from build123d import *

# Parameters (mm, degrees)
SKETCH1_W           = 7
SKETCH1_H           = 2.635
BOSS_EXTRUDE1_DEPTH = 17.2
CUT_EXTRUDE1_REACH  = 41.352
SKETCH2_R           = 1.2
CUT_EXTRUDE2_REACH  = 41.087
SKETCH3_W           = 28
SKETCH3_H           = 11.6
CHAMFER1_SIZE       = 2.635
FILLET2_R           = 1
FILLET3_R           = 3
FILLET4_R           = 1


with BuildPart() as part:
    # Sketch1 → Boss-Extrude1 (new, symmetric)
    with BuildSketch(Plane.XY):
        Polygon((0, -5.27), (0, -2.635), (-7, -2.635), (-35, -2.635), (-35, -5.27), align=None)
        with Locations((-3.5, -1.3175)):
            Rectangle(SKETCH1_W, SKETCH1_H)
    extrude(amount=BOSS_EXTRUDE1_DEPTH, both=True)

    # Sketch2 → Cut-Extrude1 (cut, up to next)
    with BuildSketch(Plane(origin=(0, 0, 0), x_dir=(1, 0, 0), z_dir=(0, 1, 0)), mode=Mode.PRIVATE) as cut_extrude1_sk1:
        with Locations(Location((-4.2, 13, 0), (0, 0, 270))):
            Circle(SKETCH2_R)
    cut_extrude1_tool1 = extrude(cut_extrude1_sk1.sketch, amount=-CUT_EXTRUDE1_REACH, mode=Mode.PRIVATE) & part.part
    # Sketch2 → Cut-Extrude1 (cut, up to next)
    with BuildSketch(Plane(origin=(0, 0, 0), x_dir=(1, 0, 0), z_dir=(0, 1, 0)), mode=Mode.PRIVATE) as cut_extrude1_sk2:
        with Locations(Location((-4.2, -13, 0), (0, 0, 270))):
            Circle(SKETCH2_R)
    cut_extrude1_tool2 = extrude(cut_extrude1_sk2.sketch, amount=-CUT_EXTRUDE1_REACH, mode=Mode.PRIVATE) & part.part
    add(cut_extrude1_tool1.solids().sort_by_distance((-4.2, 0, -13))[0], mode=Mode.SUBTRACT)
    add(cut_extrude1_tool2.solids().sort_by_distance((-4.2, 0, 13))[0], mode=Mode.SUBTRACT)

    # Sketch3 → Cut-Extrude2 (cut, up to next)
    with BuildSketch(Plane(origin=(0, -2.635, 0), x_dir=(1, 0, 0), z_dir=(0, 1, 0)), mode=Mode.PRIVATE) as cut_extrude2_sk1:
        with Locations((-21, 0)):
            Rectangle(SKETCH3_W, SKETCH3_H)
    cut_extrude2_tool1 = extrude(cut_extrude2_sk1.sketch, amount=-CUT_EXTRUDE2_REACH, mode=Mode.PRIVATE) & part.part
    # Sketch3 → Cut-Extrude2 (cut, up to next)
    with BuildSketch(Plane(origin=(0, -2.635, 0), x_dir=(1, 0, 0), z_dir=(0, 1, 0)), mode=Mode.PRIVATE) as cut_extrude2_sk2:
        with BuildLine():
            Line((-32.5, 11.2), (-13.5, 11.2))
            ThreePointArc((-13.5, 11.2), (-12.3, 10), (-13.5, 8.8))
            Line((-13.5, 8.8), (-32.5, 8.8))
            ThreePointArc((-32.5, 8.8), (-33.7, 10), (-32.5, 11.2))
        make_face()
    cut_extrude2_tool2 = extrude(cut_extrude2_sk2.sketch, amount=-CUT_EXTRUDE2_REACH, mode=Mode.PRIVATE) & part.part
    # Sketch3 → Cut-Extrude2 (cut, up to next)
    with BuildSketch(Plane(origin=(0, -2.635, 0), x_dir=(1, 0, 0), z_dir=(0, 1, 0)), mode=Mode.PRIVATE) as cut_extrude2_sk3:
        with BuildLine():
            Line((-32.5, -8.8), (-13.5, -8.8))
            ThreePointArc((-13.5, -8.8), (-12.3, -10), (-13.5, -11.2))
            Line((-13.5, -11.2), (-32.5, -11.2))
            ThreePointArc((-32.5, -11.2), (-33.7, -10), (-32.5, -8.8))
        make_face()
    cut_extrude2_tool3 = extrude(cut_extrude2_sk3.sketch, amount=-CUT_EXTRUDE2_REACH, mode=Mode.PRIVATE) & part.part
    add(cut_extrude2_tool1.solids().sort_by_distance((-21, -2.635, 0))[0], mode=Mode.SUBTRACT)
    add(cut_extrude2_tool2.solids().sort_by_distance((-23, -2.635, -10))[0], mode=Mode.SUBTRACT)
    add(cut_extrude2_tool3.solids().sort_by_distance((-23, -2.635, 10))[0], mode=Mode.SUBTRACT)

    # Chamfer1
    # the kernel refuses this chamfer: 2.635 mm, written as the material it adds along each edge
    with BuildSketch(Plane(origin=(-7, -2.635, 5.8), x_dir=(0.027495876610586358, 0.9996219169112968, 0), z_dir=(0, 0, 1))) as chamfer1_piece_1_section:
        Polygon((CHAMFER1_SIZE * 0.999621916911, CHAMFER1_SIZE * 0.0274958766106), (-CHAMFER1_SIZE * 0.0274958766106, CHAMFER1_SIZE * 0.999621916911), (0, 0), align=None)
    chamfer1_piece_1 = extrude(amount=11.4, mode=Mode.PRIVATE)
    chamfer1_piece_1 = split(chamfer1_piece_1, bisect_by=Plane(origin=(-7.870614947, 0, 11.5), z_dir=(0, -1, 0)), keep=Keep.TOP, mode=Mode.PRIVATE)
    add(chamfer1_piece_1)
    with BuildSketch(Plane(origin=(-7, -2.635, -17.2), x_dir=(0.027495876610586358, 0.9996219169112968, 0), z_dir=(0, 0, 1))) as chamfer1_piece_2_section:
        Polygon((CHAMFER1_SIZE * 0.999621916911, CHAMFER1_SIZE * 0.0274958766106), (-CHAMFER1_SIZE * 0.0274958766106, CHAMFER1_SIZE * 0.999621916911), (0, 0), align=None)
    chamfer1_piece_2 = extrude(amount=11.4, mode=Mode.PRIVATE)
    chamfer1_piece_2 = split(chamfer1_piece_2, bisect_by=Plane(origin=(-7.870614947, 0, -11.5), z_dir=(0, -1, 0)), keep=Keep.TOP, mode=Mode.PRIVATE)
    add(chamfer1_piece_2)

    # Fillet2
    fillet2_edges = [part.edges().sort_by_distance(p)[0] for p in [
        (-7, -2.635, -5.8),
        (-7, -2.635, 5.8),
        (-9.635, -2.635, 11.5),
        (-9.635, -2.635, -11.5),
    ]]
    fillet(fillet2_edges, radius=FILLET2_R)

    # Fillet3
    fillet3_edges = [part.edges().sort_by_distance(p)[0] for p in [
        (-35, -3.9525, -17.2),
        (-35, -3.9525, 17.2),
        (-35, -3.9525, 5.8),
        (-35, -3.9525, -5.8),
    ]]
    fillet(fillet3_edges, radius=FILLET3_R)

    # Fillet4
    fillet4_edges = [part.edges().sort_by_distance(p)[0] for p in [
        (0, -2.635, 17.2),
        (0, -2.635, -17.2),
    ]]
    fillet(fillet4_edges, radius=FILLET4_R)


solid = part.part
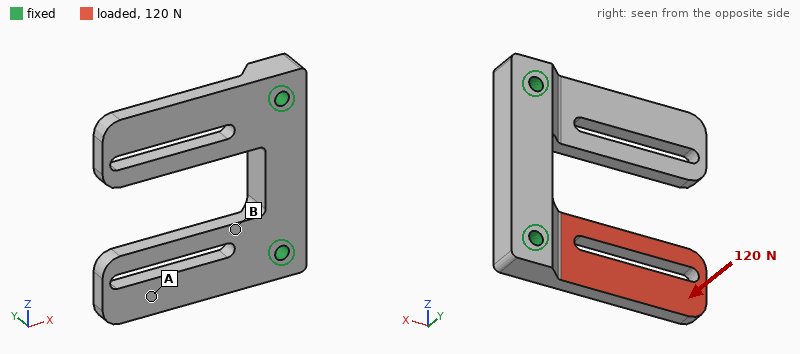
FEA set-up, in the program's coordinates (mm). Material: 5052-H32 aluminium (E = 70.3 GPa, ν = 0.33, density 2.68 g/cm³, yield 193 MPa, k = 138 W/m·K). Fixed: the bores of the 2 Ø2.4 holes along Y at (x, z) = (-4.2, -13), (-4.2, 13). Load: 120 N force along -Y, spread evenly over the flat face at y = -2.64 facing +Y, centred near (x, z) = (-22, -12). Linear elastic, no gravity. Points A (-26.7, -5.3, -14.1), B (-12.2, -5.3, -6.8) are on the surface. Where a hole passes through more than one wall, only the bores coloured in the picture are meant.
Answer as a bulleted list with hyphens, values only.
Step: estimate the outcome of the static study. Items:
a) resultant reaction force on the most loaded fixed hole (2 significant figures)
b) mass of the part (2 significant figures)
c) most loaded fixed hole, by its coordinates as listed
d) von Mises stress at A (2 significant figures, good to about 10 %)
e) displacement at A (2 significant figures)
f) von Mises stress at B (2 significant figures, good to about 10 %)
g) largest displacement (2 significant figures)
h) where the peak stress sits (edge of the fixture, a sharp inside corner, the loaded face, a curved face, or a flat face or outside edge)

- 130 N
- 7.2 g
- (-4.2, -13)
- 15 MPa
- 0.18 mm
- 100 MPa
- 0.31 mm
- the loaded face
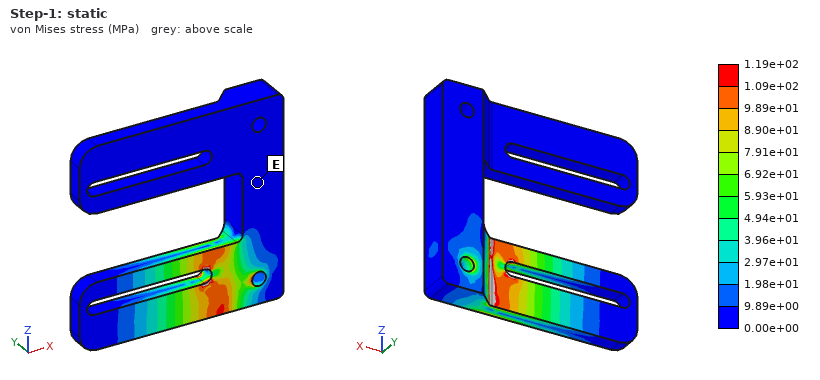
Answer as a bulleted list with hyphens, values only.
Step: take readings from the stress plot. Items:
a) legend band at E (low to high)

- 0.00e+00 to 9.89e+00 MPa
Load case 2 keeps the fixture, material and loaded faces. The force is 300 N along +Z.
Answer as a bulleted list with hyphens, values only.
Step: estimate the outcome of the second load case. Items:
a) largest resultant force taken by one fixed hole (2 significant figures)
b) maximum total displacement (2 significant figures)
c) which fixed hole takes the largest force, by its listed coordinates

- 330 N
- 0.15 mm
- (-4.2, -13)
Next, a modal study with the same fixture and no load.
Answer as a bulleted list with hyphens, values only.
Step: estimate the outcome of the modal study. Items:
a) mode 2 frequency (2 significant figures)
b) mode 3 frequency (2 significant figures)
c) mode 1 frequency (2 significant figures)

- 3100 Hz
- 6600 Hz
- 3100 Hz
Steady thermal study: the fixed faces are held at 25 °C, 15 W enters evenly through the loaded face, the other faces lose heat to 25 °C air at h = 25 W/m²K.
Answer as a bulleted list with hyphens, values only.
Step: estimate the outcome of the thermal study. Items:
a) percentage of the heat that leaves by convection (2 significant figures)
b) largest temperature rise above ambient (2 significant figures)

- 4.6 %
- 66 K
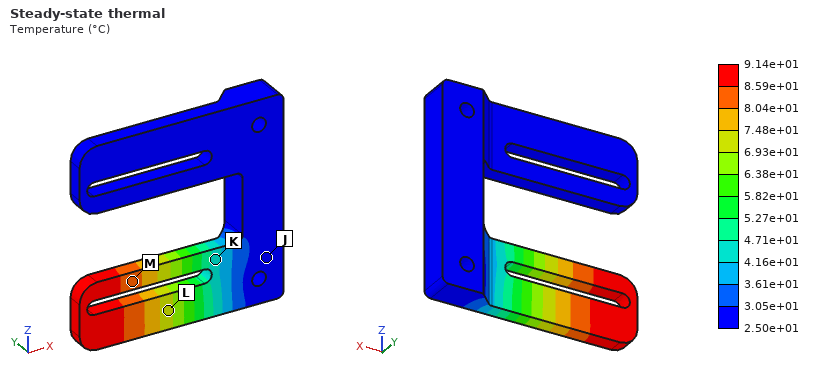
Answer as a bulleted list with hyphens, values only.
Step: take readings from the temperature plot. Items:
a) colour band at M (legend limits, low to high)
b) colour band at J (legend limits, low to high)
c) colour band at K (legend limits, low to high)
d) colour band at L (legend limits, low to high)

- 8.04e+01 to 8.59e+01 °C
- 2.50e+01 to 3.05e+01 °C
- 4.16e+01 to 4.71e+01 °C
- 6.93e+01 to 7.48e+01 °C
